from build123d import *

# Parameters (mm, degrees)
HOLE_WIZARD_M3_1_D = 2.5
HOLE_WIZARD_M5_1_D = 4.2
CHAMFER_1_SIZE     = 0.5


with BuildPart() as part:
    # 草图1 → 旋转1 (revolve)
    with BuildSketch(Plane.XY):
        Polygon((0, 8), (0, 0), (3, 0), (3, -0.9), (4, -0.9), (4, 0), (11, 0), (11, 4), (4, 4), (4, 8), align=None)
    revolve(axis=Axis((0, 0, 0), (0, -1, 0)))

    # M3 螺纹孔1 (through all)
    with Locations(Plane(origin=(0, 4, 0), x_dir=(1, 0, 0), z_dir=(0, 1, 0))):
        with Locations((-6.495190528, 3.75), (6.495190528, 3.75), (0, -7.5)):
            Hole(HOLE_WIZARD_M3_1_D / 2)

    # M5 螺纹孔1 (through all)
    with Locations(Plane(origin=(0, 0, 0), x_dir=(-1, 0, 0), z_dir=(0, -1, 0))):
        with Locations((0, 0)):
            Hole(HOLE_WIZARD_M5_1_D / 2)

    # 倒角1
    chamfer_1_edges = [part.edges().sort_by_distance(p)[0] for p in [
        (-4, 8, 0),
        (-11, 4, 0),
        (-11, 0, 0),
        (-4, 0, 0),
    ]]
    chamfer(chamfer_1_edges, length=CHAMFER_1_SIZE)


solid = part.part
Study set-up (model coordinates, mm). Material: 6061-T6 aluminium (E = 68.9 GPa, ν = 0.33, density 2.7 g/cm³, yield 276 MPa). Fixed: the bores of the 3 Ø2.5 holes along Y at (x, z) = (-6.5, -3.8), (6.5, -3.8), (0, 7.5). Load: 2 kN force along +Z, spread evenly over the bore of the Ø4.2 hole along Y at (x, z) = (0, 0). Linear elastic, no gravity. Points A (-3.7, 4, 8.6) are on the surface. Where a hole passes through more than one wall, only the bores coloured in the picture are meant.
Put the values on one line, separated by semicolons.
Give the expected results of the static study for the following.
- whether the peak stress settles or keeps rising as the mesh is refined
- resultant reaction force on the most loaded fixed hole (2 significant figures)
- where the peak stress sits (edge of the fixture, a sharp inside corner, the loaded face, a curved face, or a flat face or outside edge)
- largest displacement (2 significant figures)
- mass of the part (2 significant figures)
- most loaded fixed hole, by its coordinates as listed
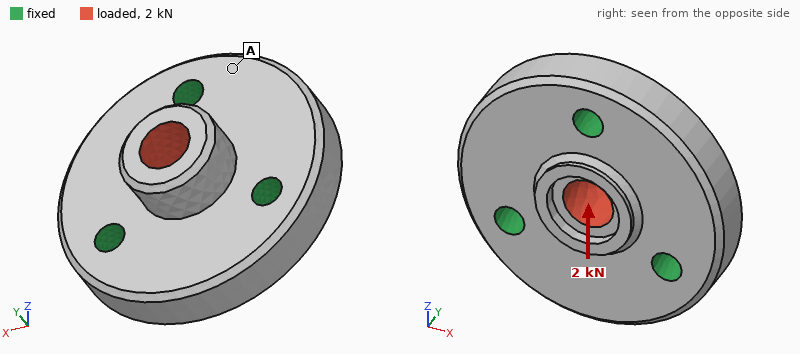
keeps rising; 800 N; edge of the fixture; 11 µm; 4.2 g; (0, 7.5)
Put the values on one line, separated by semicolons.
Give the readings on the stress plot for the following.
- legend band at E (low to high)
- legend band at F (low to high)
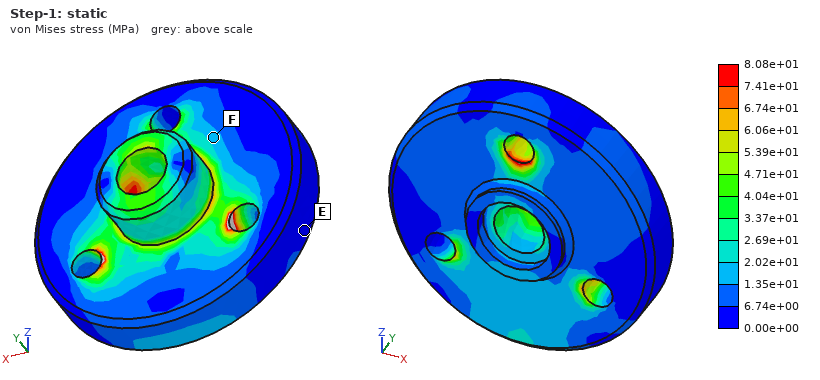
0.00e+00 to 6.74e+00 MPa; 1.35e+01 to 2.02e+01 MPa
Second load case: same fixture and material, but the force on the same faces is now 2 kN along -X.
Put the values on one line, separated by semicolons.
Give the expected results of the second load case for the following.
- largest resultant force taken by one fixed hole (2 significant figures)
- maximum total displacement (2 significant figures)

750 N; 11 µm
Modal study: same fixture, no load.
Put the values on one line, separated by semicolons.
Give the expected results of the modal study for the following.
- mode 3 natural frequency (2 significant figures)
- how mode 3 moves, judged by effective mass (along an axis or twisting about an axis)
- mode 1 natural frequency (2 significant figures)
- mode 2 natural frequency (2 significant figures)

60 kHz; along Y; 54 kHz; 54 kHz
